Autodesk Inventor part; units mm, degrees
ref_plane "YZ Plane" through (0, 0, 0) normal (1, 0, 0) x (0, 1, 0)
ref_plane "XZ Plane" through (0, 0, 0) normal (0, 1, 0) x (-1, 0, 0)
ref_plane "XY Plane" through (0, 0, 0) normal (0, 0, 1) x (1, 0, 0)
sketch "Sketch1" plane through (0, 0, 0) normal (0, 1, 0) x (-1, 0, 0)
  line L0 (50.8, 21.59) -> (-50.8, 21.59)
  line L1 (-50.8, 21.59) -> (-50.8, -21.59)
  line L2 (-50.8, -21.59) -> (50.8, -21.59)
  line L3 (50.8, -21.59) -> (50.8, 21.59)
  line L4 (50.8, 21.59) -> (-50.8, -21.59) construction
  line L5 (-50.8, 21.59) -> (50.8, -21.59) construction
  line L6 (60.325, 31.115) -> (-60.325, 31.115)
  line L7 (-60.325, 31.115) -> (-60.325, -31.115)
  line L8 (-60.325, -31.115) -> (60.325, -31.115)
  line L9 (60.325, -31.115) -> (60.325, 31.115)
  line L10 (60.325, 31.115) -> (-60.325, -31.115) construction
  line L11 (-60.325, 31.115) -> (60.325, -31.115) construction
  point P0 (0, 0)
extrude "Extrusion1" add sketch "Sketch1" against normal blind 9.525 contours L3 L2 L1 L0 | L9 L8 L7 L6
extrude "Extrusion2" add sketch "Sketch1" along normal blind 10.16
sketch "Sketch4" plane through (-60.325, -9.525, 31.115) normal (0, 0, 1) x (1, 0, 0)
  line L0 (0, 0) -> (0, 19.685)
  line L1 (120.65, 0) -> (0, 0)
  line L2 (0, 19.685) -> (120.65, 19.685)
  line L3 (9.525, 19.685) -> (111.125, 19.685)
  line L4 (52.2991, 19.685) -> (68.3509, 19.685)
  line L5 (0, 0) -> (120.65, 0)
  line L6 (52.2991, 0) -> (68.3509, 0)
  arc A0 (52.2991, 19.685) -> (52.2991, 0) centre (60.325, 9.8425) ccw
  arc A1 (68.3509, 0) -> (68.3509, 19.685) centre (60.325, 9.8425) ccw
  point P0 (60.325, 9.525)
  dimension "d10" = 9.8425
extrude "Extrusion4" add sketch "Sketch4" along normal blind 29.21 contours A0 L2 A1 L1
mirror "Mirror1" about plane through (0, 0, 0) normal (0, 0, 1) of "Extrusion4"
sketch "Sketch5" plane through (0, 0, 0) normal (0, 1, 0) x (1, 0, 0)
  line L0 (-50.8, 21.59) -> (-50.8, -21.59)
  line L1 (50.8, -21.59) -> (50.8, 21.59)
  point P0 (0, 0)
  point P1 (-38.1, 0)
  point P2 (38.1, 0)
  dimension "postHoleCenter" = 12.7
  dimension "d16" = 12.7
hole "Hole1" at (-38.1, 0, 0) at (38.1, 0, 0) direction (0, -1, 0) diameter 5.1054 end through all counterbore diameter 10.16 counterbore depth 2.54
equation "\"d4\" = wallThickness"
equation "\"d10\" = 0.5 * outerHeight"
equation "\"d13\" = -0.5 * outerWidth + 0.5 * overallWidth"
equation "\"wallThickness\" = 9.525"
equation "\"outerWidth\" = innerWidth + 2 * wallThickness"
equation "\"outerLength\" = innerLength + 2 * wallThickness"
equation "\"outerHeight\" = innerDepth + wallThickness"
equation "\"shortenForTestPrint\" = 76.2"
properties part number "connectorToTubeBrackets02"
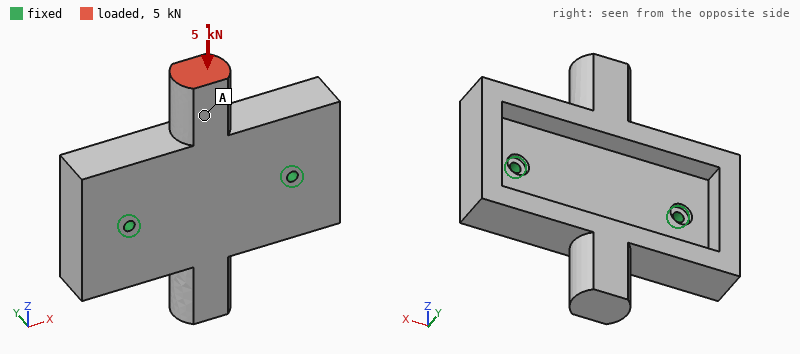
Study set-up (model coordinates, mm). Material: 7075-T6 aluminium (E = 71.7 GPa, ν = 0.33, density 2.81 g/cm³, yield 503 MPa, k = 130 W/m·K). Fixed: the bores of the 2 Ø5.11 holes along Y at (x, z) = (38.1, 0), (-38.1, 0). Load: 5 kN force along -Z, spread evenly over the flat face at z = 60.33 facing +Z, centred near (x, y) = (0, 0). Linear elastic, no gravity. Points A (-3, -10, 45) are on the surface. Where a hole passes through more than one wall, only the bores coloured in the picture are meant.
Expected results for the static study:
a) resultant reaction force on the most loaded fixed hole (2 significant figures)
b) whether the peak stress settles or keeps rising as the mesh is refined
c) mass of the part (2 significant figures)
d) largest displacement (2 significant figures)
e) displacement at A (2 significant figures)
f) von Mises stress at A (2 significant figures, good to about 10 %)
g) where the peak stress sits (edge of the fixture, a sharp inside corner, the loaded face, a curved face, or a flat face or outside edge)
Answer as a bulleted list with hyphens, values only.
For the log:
- 2.5 kN
- keeps rising
- 360 g
- 0.13 mm
- 0.086 mm
- 11 MPa
- edge of the fixture
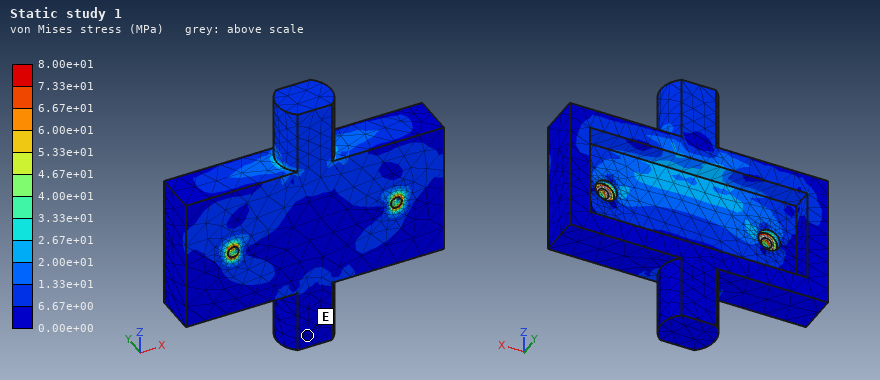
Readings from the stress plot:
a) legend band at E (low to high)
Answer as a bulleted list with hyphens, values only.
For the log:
- 0.00e+00 to 6.67e+00 MPa
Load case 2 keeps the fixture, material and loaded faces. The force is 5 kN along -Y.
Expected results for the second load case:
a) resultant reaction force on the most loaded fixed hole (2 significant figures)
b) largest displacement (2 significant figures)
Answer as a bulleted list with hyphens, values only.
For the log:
- 2.7 kN
- 1.3 mm
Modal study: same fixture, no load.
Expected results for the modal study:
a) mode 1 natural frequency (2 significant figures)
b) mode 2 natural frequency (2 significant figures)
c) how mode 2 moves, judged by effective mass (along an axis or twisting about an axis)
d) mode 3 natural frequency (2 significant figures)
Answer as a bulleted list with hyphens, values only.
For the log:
- 1500 Hz
- 2800 Hz
- along Y
- 4400 Hz
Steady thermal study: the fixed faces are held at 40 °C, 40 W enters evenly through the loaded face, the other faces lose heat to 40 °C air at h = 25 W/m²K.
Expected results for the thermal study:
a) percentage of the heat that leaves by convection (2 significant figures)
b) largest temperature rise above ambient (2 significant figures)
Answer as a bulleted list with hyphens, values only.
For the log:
- 14 %
- 39 K
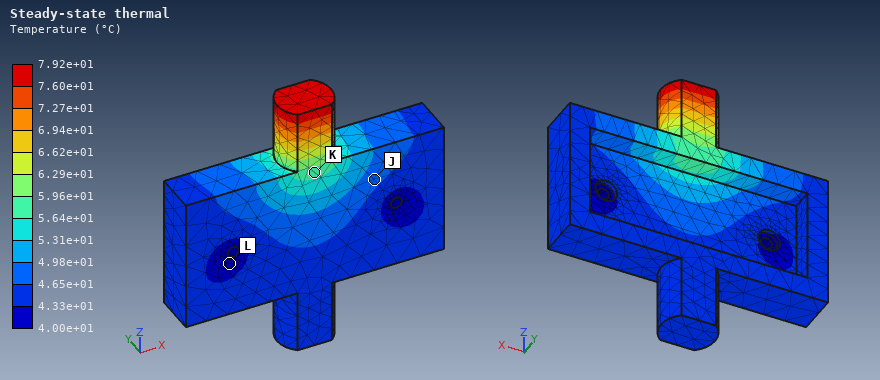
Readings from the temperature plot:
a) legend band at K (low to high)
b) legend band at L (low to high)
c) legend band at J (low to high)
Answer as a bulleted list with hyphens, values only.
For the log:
- 5.64e+01 to 5.96e+01 °C
- 4.00e+01 to 4.33e+01 °C
- 4.65e+01 to 4.98e+01 °C
